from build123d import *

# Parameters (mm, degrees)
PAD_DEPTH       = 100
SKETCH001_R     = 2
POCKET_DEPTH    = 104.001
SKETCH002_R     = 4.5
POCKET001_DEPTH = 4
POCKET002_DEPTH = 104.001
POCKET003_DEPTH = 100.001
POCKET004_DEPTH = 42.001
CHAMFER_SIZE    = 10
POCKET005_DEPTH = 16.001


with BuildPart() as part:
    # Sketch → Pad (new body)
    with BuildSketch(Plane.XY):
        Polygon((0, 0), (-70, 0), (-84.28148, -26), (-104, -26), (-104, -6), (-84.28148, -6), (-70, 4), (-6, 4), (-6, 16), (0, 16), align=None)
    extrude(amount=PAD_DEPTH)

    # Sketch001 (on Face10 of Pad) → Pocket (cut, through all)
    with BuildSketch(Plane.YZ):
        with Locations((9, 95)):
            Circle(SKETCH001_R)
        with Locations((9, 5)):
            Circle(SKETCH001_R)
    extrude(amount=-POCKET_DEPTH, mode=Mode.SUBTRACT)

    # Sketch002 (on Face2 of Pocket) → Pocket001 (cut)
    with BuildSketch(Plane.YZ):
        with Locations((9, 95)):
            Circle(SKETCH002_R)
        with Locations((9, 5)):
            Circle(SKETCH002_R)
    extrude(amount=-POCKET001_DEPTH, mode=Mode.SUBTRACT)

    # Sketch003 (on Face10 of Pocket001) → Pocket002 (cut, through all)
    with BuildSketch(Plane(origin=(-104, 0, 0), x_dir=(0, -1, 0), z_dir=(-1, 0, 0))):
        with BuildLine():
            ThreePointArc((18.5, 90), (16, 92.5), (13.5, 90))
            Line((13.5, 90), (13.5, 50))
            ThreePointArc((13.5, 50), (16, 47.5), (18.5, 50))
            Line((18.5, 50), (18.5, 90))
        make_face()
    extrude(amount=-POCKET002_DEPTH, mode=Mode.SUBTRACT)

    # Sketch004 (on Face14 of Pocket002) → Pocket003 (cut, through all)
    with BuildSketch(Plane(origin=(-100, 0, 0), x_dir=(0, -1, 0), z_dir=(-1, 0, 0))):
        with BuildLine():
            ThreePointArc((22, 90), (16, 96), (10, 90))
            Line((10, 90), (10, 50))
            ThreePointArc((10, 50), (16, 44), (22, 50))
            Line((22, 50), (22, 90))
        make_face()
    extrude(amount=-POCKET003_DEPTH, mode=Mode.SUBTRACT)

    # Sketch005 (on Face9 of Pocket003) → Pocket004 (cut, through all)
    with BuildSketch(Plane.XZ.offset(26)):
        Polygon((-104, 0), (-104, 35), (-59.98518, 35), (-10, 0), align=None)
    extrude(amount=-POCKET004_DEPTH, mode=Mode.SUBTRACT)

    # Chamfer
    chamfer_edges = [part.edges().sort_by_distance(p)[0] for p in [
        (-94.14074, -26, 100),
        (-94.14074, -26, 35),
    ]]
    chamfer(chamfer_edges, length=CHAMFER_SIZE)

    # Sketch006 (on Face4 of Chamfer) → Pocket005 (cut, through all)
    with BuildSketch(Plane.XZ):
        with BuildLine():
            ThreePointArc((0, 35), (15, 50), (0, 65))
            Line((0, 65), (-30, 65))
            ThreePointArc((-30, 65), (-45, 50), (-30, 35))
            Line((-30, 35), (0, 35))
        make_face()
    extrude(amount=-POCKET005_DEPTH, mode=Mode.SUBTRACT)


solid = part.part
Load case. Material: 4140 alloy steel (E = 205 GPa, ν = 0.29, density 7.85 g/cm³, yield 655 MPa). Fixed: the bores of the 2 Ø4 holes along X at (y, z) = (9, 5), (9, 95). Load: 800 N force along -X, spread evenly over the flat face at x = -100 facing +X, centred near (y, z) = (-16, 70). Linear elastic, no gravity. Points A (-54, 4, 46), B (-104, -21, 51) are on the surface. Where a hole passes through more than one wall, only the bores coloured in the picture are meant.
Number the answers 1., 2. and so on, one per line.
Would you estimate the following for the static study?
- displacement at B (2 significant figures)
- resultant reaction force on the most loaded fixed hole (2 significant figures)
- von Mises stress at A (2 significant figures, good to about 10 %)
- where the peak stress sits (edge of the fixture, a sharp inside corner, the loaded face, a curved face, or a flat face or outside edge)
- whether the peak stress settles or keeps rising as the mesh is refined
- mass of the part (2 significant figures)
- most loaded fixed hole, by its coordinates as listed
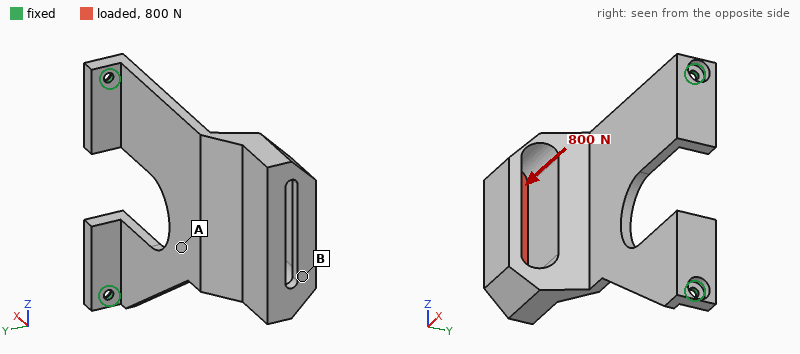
1. 1.6 mm
2. 610 N
3. 65 MPa
4. edge of the fixture
5. keeps rising
6. 340 g
7. (9, 95)
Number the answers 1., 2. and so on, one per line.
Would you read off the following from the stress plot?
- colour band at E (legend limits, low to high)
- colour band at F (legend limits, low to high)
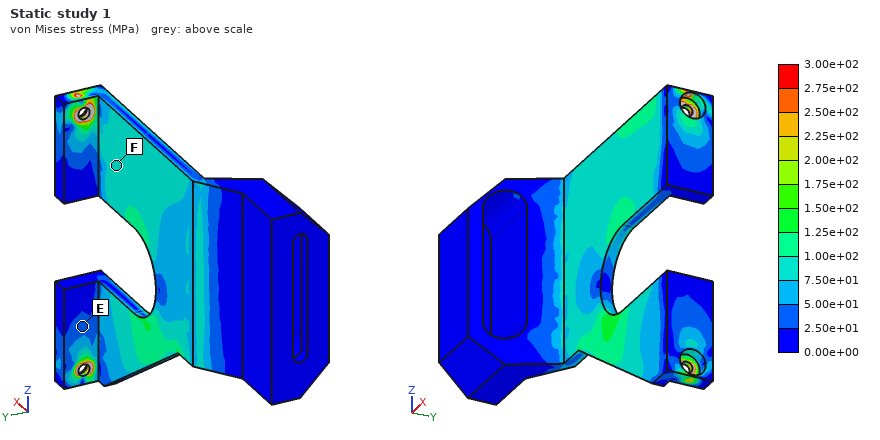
1. 2.50e+01 to 5.00e+01 MPa
2. 7.50e+01 to 1.00e+02 MPa
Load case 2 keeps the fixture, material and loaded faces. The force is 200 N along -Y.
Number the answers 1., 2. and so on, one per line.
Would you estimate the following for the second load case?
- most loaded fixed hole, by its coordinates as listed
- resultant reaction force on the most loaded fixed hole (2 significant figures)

1. (9, 95)
2. 120 N
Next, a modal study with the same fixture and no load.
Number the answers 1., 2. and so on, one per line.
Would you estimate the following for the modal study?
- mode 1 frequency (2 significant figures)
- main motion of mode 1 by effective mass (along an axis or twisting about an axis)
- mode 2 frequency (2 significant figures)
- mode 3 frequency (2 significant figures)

1. 160 Hz
2. along Y
3. 680 Hz
4. 1200 Hz
